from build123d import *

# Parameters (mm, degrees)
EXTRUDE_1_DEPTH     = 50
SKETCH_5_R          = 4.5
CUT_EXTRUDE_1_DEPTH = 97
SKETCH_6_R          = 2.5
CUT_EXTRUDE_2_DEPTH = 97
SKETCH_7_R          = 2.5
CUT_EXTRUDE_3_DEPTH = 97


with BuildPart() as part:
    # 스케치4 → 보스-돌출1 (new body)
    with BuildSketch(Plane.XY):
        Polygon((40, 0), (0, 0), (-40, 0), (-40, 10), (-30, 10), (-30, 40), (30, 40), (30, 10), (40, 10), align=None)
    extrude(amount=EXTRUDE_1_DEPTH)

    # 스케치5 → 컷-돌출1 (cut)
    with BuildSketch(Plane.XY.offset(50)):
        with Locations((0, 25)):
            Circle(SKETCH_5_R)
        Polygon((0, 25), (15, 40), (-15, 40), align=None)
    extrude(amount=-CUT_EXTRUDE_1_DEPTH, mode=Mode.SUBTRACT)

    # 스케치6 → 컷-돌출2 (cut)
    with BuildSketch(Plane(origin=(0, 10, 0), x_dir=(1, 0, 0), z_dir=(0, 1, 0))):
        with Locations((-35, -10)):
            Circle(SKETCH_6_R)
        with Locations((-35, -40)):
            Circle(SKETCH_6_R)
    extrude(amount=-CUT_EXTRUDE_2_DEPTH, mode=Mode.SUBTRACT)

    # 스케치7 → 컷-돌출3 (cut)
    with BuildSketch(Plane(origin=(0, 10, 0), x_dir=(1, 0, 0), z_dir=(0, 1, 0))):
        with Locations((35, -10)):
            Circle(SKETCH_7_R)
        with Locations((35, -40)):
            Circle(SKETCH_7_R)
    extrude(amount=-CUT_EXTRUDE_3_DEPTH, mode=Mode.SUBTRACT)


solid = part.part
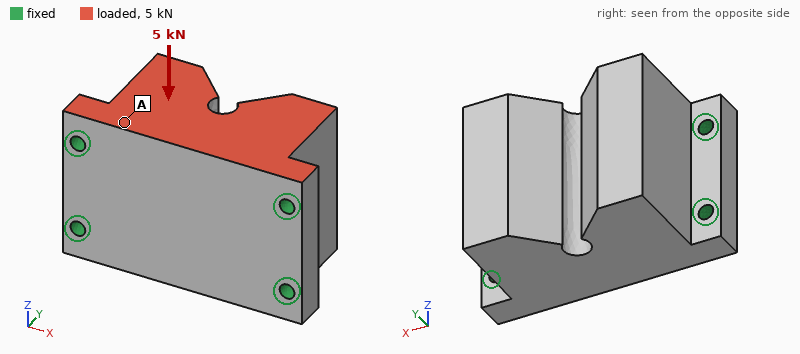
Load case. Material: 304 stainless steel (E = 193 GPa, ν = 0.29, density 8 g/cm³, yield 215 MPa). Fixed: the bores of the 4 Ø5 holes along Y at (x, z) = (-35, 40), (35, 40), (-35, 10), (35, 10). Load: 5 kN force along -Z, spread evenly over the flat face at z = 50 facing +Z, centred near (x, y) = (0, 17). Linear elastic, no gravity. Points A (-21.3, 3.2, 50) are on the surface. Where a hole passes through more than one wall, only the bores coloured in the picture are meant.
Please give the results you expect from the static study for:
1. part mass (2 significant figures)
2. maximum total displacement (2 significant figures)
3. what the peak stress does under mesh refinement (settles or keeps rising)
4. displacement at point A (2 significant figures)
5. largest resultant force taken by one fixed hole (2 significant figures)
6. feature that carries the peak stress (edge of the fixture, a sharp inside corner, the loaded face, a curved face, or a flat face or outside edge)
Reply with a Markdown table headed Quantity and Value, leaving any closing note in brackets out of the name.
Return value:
| Quantity | Value |
|---|---|
| part mass | 920 g |
| maximum total displacement | 4.0 µm |
| what the peak stress does under mesh refinement | keeps rising |
| displacement at point A | 1.8 µm |
| largest resultant force taken by one fixed hole | 1.7 kN |
| feature that carries the peak stress | edge of the fixture |
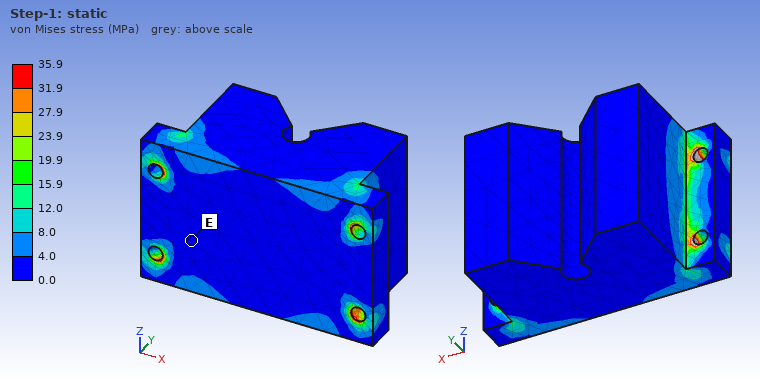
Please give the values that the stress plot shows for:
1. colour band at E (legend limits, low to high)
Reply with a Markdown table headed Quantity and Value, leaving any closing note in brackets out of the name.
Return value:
| Quantity | Value |
|---|---|
| colour band at E | 0.0 to 4.0 MPa |
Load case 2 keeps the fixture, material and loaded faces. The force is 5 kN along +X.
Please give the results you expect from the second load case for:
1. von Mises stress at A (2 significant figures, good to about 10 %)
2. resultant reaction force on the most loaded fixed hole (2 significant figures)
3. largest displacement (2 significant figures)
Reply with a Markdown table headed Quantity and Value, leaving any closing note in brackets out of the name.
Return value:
| Quantity | Value |
|---|---|
| von Mises stress at A | 6.4 MPa |
| resultant reaction force on the most loaded fixed hole | 2.0 kN |
| largest displacement | 2.9 µm |
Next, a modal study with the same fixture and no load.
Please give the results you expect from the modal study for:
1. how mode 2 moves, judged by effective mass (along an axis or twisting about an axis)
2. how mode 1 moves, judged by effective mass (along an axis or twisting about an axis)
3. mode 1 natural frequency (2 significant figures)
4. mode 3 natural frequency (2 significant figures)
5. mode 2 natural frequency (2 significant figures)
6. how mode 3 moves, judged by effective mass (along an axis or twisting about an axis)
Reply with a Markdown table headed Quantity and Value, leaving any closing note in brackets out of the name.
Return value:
| Quantity | Value |
|---|---|
| how mode 2 moves, judged by effective mass | along Y |
| how mode 1 moves, judged by effective mass | along Z |
| mode 1 natural frequency | 6800 Hz |
| mode 3 natural frequency | 12 kHz |
| mode 2 natural frequency | 8200 Hz |
| how mode 3 moves, judged by effective mass | along X |
